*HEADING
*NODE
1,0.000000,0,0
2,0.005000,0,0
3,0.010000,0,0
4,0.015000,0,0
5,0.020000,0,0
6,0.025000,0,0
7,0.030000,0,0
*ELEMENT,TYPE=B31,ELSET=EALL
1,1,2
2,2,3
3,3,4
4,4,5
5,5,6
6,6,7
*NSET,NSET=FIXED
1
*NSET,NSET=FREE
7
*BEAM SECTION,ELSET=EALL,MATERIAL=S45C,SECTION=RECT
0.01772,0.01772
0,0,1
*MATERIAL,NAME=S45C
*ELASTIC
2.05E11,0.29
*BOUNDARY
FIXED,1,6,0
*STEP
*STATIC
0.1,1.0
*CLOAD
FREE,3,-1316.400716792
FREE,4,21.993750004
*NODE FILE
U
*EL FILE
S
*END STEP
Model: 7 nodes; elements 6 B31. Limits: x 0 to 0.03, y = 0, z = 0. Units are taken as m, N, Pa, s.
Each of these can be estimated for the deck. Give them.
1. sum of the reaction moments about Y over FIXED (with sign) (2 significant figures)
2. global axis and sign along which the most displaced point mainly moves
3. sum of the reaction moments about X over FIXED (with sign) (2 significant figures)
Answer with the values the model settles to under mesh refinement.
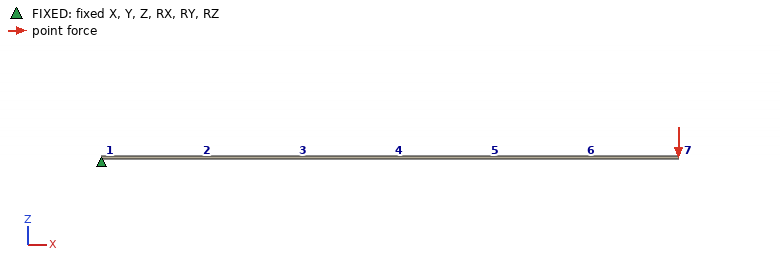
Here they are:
-39 N·m
-Z
-22 N·m
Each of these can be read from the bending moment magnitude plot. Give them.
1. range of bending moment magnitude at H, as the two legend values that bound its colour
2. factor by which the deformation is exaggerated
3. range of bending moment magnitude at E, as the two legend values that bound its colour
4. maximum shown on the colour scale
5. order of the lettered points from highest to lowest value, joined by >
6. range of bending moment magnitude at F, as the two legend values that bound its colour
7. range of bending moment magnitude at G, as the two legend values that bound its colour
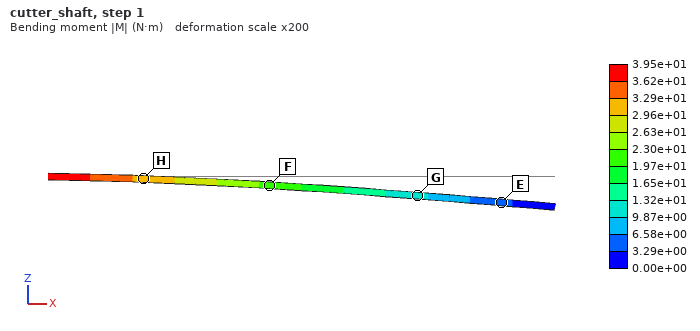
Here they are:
2.96e+01 to 3.29e+01 N·m
200
3.29e+00 to 6.58e+00 N·m
3.95e+01 N·m
H > F > G > E
1.97e+01 to 2.30e+01 N·m
9.87e+00 to 1.32e+01 N·m
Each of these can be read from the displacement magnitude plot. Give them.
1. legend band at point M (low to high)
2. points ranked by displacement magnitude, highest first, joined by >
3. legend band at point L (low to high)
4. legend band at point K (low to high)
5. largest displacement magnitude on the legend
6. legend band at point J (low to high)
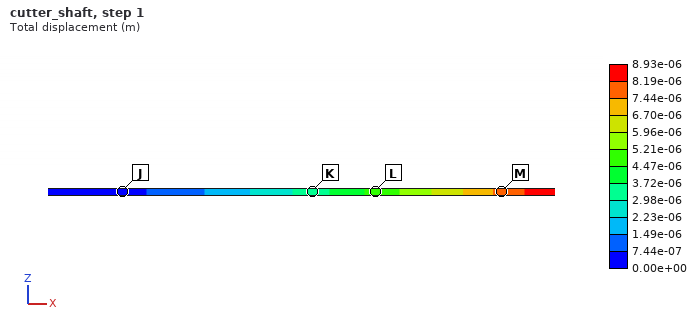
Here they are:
7.44e-06 to 8.19e-06 m
M > L > K > J
4.47e-06 to 5.21e-06 m
2.98e-06 to 3.72e-06 m
8.93e-06 m
0.00e+00 to 7.44e-07 m
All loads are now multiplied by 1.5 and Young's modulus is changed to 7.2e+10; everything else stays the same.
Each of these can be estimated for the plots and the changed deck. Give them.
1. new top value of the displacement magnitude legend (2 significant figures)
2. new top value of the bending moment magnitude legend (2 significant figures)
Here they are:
3.8e-05 m
59 N·m
